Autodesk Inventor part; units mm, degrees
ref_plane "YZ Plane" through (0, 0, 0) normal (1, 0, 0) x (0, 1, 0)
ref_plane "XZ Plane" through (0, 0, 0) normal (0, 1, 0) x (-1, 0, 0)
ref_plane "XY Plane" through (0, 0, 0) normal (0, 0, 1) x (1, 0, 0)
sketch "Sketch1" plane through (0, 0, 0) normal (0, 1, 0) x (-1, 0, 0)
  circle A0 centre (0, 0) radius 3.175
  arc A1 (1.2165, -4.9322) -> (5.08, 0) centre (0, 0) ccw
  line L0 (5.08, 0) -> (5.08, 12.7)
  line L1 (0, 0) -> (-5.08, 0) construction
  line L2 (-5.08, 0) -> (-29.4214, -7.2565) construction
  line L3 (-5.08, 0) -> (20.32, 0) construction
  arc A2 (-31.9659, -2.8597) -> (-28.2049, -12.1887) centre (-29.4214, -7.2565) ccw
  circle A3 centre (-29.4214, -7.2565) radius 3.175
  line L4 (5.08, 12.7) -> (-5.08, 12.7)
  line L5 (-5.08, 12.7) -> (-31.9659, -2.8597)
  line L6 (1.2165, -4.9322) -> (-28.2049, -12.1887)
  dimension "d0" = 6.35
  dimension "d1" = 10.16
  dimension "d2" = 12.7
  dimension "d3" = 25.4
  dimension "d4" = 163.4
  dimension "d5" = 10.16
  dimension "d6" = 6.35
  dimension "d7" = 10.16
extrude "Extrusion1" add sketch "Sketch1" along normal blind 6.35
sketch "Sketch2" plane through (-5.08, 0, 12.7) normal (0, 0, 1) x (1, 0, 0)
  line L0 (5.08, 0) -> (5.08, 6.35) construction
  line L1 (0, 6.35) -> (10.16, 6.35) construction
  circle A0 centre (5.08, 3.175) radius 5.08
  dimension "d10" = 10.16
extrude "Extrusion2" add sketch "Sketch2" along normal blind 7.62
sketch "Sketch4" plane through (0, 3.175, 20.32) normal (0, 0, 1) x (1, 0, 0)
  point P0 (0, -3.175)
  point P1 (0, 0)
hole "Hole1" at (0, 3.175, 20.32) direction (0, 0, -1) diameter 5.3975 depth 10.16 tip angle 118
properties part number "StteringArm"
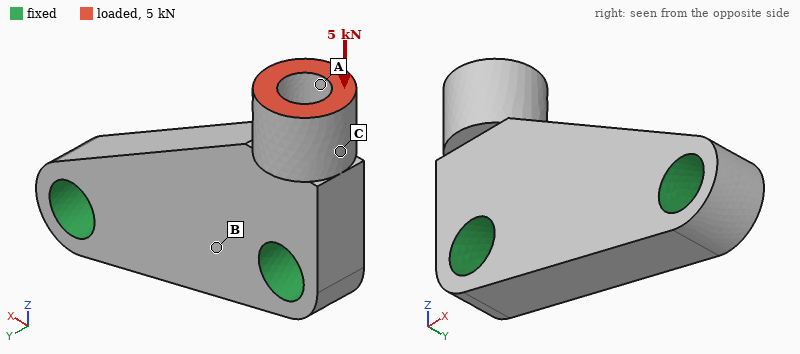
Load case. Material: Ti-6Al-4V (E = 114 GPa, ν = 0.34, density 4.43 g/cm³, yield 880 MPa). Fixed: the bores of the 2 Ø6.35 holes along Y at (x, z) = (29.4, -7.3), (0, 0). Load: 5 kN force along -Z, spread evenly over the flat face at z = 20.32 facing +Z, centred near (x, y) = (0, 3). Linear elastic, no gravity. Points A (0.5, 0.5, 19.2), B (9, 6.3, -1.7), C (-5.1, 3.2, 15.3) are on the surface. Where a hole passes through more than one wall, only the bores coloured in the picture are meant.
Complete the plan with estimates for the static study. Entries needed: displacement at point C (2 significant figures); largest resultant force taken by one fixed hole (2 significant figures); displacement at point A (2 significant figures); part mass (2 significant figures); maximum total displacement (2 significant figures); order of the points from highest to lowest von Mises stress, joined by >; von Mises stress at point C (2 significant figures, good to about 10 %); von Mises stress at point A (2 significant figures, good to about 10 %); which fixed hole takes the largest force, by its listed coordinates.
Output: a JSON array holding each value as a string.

["14 µm", "4.8 kN", "17 µm", "16 g", "19 µm", "C > A > B", "110 MPa", "74 MPa", "(0, 0)"]
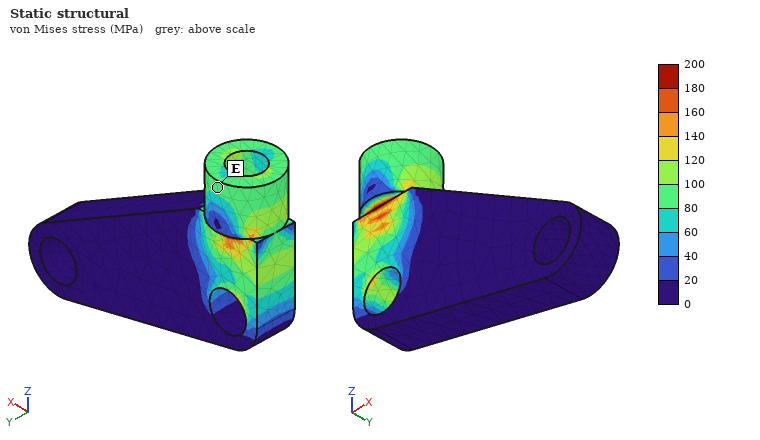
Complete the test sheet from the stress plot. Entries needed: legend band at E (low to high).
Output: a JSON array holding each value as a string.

["80 to 100 MPa"]
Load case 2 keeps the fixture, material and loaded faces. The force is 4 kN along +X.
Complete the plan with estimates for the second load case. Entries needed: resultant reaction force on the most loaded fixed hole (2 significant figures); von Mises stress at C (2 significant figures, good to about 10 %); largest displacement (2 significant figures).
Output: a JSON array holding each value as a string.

["3.2 kN", "210 MPa", "0.12 mm"]
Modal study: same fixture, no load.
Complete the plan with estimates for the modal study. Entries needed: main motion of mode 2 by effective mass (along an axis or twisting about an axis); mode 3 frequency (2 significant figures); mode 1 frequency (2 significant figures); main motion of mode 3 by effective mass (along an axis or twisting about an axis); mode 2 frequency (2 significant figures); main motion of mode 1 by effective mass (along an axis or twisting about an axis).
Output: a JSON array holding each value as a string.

["along X", "29 kHz", "16 kHz", "along Y", "28 kHz", "along Y"]
